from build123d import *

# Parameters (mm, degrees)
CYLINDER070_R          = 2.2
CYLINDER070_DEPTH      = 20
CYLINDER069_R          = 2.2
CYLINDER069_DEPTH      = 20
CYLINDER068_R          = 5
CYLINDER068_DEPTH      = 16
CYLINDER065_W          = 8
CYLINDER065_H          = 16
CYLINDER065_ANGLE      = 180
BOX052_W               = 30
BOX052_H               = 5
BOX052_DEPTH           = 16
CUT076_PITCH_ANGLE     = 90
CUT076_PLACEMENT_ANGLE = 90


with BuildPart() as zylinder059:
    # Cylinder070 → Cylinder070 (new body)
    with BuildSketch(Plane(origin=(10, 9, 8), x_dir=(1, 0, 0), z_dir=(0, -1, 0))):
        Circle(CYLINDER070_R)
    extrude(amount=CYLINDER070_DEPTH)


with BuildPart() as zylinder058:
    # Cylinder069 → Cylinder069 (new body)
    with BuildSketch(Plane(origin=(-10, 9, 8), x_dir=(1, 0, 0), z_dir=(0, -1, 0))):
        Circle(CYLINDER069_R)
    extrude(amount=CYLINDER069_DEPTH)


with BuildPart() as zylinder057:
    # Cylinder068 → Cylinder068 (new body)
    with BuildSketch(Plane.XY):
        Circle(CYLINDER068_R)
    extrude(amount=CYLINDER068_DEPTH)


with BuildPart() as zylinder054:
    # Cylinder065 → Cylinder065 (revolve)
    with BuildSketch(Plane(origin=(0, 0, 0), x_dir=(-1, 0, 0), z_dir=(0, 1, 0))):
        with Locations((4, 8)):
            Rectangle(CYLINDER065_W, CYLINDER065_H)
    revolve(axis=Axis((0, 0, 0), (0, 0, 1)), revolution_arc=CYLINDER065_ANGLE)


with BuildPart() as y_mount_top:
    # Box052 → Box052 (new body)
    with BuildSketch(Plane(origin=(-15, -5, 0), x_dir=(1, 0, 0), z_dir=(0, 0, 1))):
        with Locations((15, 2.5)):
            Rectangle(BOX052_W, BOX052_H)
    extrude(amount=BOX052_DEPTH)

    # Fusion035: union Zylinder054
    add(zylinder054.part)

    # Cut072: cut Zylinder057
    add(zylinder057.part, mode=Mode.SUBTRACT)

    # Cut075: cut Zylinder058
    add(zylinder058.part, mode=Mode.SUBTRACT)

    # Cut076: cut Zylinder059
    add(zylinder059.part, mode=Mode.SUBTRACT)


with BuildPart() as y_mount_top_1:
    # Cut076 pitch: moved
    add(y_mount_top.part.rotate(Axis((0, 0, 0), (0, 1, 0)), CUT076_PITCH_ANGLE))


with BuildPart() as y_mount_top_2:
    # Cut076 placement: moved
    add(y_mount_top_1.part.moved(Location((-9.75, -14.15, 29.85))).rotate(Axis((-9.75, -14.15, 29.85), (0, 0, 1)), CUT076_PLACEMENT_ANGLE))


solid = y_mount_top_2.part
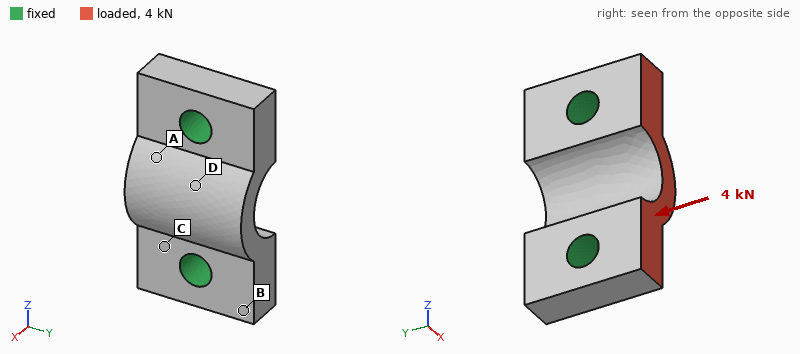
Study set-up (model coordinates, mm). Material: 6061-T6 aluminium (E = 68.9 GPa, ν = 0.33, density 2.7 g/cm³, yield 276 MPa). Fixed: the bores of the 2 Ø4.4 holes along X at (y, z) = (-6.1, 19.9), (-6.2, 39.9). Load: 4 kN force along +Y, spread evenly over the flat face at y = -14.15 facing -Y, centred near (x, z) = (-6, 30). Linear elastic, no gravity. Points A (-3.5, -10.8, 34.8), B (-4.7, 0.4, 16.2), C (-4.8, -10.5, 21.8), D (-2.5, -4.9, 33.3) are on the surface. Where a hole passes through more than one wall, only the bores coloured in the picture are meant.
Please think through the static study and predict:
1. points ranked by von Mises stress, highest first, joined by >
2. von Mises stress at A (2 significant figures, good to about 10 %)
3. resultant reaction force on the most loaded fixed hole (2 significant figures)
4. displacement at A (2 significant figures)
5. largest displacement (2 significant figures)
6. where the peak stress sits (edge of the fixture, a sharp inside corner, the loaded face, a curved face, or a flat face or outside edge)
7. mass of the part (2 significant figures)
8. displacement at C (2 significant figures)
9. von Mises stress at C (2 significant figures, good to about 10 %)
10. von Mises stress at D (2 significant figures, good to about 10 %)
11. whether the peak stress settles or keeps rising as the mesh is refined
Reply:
C > A > D > B
35 MPa
2.0 kN
7.7 µm
14 µm
edge of the fixture
5.5 g
3.4 µm
52 MPa
22 MPa
keeps rising
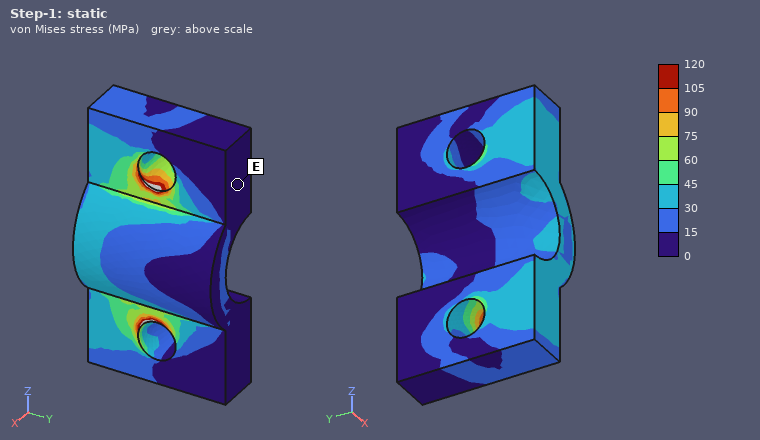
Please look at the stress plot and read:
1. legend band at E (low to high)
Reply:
0 to 15 MPa
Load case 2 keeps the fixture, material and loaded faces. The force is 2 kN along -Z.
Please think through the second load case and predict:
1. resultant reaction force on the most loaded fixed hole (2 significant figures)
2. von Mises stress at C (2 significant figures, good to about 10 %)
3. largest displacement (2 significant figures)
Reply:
1.1 kN
51 MPa
11 µm
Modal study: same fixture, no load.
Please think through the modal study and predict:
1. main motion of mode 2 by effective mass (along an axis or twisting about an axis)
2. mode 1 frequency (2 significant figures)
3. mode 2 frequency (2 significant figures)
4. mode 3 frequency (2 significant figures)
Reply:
along X
40 kHz
56 kHz
62 kHz
